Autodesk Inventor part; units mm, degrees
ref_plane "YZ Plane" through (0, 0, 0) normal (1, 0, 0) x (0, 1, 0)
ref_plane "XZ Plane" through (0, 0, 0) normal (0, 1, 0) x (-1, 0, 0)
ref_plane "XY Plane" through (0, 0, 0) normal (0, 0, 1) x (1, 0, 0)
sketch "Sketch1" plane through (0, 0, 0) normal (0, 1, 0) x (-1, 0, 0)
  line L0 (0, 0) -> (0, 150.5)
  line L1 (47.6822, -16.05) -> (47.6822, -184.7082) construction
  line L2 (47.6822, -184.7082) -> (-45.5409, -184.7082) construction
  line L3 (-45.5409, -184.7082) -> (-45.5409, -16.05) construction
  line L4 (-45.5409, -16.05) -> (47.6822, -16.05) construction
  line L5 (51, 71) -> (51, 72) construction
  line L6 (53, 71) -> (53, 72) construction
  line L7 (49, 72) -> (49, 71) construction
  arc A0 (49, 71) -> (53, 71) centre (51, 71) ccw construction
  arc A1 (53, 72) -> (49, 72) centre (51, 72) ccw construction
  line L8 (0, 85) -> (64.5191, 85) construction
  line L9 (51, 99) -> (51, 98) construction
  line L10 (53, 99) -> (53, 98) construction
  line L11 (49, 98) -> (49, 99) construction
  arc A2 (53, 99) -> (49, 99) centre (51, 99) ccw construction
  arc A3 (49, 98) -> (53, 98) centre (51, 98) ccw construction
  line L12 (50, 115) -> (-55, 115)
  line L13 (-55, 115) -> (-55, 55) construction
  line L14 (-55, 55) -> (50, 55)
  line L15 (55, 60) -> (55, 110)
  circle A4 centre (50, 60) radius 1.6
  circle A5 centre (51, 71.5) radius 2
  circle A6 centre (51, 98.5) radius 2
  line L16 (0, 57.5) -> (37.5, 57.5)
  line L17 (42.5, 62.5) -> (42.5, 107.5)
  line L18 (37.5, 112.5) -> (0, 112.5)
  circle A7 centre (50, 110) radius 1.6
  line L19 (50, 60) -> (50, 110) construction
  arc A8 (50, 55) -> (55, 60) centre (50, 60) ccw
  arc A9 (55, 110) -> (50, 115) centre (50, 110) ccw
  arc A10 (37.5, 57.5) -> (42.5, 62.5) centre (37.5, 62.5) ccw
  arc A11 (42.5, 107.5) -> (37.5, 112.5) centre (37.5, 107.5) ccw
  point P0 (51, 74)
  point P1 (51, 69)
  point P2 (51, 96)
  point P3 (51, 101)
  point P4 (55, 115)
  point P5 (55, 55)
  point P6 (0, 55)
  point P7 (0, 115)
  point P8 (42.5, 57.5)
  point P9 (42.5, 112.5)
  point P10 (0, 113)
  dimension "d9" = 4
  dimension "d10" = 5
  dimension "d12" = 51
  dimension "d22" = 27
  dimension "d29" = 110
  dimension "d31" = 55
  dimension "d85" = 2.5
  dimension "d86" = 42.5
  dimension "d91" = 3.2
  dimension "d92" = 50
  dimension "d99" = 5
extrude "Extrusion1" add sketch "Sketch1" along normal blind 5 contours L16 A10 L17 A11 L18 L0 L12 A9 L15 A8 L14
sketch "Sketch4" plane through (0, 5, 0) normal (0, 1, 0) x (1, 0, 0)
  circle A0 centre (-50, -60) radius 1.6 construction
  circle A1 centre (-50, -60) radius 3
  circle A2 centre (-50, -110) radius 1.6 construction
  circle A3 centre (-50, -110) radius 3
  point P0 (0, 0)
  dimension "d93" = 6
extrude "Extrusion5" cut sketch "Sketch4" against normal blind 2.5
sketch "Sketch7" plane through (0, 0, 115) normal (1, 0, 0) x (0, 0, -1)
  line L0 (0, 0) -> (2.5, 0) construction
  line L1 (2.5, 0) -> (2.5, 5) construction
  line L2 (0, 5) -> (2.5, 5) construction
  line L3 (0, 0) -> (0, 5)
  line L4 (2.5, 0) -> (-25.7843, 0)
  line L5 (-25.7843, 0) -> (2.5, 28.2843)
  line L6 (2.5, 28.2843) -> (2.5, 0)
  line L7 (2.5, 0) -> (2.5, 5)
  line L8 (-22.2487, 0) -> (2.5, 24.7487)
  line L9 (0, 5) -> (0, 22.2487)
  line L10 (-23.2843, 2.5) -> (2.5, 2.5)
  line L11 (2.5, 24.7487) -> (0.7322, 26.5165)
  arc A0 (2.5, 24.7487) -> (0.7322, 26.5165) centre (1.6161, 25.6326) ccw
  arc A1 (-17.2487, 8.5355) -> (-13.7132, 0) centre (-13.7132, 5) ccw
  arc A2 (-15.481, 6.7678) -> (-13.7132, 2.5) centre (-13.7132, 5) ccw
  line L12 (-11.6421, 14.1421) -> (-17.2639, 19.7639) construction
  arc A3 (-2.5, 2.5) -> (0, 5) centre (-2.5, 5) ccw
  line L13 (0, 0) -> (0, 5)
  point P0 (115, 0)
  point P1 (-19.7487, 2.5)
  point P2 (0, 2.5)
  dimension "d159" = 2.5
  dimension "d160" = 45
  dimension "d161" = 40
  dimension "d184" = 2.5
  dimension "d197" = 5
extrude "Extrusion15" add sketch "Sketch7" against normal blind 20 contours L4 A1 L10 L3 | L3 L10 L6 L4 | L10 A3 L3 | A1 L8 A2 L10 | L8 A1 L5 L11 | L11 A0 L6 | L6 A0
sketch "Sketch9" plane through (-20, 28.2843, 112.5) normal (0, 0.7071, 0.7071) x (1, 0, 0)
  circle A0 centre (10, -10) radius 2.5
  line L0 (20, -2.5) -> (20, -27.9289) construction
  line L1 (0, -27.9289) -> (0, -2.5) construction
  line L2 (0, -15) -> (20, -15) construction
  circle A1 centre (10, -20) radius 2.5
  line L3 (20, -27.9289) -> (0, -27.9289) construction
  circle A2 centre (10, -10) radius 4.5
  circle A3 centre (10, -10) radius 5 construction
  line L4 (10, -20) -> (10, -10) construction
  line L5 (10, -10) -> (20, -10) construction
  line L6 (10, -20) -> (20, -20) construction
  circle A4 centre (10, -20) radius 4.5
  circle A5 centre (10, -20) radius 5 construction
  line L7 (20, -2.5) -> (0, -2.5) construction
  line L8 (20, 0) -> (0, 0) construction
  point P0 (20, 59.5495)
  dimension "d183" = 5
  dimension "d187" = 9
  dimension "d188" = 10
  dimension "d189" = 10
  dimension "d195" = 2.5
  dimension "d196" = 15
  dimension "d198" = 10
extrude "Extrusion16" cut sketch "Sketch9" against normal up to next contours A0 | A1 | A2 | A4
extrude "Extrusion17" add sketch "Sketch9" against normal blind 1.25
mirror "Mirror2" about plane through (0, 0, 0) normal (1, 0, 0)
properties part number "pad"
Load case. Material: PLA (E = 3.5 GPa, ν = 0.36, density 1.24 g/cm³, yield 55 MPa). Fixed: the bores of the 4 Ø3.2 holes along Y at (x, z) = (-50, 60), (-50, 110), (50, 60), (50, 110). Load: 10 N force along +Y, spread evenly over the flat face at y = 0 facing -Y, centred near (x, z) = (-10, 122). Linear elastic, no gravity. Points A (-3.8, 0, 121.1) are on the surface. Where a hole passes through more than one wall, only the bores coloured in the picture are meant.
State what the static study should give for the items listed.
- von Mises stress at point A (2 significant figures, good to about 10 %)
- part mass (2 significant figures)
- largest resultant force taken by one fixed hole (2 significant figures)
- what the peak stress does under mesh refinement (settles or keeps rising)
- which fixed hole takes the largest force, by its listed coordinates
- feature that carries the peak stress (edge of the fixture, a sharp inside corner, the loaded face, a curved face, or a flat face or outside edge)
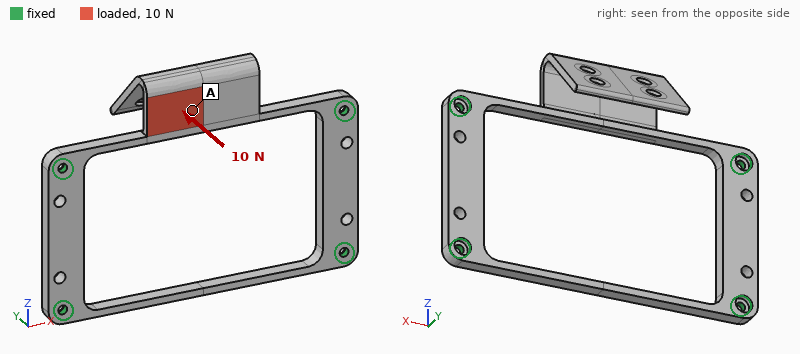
1.8 MPa
17 g
8.0 N
keeps rising
(-50, 110)
edge of the fixture
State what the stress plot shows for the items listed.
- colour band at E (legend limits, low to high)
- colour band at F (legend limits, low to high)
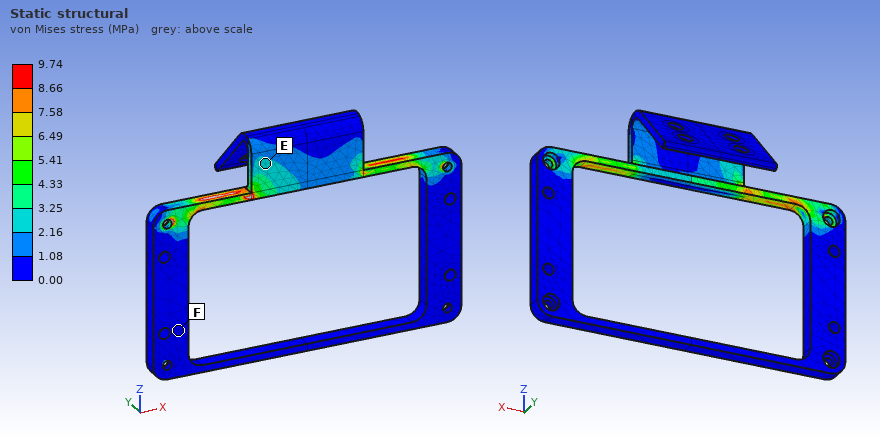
2.16 to 3.25 MPa
0.00 to 1.08 MPa
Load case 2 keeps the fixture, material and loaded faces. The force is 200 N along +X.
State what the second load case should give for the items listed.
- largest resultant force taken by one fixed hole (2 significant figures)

100 N
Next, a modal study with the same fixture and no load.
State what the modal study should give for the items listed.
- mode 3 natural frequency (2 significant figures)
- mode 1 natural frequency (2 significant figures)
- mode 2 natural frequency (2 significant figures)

540 Hz
170 Hz
350 Hz
